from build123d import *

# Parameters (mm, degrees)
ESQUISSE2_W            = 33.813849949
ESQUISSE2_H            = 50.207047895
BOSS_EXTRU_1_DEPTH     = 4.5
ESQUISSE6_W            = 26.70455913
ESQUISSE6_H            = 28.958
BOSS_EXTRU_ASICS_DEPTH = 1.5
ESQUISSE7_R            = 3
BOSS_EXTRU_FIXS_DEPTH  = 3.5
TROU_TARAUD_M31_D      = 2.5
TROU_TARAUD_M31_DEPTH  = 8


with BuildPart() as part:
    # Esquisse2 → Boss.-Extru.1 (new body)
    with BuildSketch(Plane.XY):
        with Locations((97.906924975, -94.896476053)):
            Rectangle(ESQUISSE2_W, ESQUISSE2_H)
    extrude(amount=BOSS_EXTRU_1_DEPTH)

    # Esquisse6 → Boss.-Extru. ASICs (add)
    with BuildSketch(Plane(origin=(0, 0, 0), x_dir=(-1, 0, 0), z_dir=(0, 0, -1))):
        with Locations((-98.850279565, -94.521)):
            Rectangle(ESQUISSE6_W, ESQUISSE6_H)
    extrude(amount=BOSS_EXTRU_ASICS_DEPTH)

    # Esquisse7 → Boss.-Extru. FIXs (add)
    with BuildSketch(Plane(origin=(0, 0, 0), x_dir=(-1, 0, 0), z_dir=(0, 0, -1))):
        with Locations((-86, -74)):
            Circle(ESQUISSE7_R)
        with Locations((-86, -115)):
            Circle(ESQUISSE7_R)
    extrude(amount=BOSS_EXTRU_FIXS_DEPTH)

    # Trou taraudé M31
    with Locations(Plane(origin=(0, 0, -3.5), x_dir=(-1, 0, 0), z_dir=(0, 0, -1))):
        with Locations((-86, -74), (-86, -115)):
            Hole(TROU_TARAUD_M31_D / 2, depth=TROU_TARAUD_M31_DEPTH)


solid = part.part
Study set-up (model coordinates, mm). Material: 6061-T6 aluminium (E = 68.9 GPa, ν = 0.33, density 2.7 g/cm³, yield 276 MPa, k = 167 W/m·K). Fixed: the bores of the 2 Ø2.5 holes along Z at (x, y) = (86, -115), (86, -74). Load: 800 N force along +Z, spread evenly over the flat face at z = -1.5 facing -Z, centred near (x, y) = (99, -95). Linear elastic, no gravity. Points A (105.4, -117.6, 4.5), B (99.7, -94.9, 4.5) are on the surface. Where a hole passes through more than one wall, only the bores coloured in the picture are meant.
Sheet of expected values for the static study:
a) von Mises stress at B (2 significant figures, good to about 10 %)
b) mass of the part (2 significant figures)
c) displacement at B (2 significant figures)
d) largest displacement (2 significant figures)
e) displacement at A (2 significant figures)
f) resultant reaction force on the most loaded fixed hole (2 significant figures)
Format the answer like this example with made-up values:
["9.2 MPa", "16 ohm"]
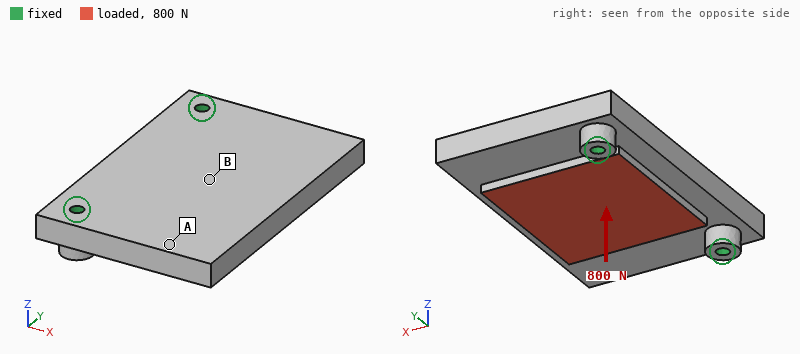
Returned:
["23 MPa", "24 g", "0.062 mm", "0.13 mm", "0.064 mm", "410 N"]
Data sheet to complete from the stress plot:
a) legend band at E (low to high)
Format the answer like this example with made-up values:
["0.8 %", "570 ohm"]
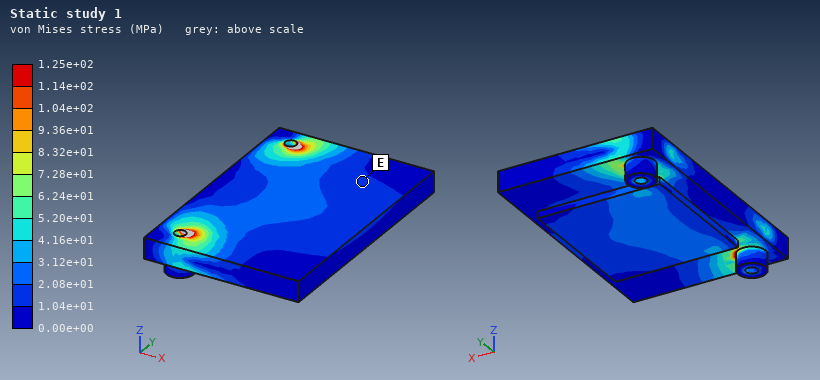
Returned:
["1.04e+01 to 2.08e+01 MPa"]
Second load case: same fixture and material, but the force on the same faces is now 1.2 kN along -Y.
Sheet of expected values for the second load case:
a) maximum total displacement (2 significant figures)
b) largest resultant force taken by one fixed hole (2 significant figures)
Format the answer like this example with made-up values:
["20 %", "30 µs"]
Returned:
["11 µm", "720 N"]
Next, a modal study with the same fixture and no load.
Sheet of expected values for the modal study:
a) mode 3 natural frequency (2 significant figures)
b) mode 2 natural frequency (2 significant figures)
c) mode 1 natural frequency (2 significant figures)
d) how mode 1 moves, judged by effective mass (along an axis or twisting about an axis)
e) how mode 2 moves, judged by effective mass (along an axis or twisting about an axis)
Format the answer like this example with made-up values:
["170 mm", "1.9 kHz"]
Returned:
["13 kHz", "8300 Hz", "3400 Hz", "along Z", "twisting about X"]
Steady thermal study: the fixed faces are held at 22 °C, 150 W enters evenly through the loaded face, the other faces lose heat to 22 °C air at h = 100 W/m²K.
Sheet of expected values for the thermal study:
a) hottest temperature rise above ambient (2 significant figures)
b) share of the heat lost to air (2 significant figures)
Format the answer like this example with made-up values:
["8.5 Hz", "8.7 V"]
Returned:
["82 K", "12 %"]
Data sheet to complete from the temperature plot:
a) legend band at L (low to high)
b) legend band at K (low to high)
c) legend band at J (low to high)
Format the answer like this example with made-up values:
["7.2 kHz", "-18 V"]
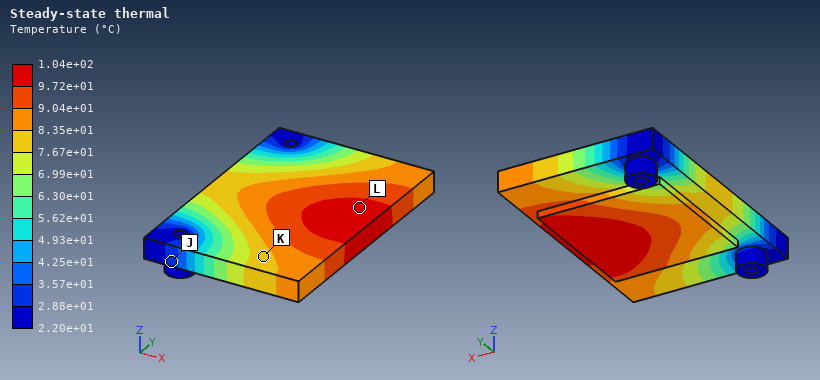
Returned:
["9.72e+01 to 1.04e+02 °C", "7.67e+01 to 8.35e+01 °C", "2.88e+01 to 3.57e+01 °C"]
